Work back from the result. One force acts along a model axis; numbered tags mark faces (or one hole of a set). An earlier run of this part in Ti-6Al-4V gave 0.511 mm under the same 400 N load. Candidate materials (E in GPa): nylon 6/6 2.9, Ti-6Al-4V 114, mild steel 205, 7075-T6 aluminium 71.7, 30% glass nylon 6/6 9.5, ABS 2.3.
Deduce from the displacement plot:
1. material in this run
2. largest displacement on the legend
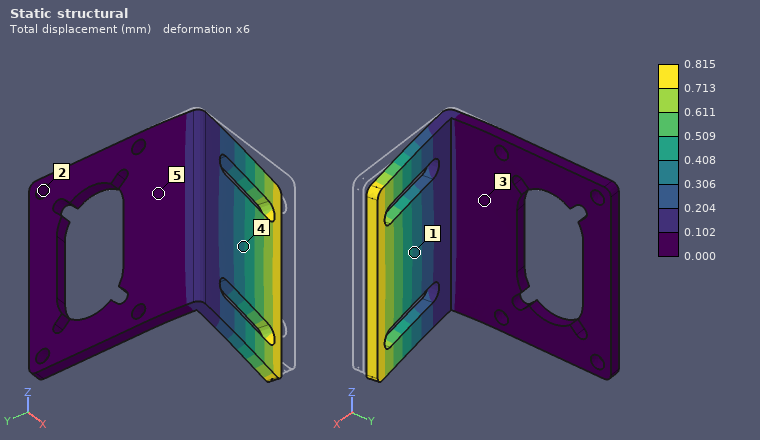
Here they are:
7075-T6 aluminium
0.815 mm
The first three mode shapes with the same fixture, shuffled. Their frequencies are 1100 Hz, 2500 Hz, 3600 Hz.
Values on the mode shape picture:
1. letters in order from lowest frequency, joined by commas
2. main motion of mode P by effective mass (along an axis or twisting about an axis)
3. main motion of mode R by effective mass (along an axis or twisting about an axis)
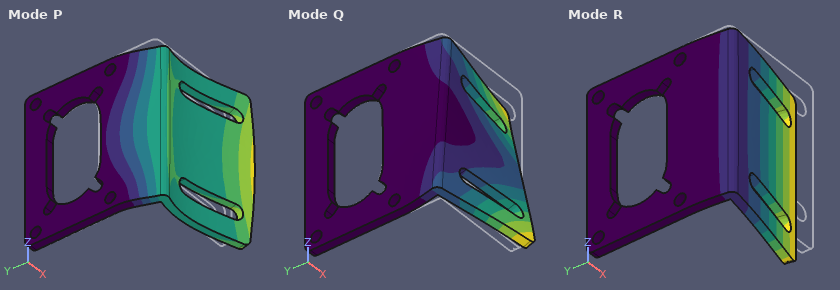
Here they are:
R, Q, P
along X
along Y
